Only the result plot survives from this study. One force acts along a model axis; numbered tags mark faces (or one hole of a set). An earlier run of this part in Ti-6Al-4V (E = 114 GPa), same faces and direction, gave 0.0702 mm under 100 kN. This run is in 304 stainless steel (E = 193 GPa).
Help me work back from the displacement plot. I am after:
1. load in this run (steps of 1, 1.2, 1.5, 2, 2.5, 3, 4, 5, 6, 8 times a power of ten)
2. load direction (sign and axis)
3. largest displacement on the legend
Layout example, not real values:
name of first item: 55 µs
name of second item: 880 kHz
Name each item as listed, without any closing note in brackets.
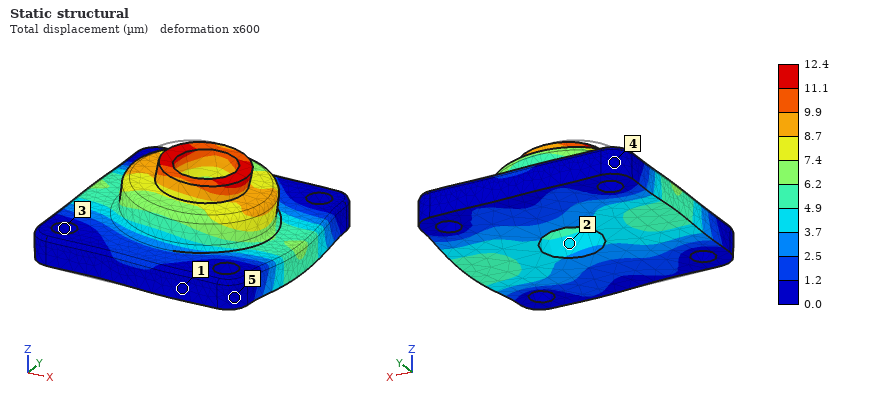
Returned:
load in this run: 30 kN
load direction: +X
largest displacement on the legend: 12.4 µm
